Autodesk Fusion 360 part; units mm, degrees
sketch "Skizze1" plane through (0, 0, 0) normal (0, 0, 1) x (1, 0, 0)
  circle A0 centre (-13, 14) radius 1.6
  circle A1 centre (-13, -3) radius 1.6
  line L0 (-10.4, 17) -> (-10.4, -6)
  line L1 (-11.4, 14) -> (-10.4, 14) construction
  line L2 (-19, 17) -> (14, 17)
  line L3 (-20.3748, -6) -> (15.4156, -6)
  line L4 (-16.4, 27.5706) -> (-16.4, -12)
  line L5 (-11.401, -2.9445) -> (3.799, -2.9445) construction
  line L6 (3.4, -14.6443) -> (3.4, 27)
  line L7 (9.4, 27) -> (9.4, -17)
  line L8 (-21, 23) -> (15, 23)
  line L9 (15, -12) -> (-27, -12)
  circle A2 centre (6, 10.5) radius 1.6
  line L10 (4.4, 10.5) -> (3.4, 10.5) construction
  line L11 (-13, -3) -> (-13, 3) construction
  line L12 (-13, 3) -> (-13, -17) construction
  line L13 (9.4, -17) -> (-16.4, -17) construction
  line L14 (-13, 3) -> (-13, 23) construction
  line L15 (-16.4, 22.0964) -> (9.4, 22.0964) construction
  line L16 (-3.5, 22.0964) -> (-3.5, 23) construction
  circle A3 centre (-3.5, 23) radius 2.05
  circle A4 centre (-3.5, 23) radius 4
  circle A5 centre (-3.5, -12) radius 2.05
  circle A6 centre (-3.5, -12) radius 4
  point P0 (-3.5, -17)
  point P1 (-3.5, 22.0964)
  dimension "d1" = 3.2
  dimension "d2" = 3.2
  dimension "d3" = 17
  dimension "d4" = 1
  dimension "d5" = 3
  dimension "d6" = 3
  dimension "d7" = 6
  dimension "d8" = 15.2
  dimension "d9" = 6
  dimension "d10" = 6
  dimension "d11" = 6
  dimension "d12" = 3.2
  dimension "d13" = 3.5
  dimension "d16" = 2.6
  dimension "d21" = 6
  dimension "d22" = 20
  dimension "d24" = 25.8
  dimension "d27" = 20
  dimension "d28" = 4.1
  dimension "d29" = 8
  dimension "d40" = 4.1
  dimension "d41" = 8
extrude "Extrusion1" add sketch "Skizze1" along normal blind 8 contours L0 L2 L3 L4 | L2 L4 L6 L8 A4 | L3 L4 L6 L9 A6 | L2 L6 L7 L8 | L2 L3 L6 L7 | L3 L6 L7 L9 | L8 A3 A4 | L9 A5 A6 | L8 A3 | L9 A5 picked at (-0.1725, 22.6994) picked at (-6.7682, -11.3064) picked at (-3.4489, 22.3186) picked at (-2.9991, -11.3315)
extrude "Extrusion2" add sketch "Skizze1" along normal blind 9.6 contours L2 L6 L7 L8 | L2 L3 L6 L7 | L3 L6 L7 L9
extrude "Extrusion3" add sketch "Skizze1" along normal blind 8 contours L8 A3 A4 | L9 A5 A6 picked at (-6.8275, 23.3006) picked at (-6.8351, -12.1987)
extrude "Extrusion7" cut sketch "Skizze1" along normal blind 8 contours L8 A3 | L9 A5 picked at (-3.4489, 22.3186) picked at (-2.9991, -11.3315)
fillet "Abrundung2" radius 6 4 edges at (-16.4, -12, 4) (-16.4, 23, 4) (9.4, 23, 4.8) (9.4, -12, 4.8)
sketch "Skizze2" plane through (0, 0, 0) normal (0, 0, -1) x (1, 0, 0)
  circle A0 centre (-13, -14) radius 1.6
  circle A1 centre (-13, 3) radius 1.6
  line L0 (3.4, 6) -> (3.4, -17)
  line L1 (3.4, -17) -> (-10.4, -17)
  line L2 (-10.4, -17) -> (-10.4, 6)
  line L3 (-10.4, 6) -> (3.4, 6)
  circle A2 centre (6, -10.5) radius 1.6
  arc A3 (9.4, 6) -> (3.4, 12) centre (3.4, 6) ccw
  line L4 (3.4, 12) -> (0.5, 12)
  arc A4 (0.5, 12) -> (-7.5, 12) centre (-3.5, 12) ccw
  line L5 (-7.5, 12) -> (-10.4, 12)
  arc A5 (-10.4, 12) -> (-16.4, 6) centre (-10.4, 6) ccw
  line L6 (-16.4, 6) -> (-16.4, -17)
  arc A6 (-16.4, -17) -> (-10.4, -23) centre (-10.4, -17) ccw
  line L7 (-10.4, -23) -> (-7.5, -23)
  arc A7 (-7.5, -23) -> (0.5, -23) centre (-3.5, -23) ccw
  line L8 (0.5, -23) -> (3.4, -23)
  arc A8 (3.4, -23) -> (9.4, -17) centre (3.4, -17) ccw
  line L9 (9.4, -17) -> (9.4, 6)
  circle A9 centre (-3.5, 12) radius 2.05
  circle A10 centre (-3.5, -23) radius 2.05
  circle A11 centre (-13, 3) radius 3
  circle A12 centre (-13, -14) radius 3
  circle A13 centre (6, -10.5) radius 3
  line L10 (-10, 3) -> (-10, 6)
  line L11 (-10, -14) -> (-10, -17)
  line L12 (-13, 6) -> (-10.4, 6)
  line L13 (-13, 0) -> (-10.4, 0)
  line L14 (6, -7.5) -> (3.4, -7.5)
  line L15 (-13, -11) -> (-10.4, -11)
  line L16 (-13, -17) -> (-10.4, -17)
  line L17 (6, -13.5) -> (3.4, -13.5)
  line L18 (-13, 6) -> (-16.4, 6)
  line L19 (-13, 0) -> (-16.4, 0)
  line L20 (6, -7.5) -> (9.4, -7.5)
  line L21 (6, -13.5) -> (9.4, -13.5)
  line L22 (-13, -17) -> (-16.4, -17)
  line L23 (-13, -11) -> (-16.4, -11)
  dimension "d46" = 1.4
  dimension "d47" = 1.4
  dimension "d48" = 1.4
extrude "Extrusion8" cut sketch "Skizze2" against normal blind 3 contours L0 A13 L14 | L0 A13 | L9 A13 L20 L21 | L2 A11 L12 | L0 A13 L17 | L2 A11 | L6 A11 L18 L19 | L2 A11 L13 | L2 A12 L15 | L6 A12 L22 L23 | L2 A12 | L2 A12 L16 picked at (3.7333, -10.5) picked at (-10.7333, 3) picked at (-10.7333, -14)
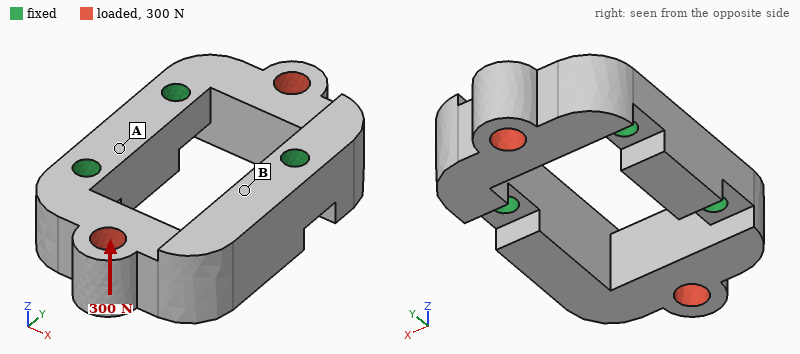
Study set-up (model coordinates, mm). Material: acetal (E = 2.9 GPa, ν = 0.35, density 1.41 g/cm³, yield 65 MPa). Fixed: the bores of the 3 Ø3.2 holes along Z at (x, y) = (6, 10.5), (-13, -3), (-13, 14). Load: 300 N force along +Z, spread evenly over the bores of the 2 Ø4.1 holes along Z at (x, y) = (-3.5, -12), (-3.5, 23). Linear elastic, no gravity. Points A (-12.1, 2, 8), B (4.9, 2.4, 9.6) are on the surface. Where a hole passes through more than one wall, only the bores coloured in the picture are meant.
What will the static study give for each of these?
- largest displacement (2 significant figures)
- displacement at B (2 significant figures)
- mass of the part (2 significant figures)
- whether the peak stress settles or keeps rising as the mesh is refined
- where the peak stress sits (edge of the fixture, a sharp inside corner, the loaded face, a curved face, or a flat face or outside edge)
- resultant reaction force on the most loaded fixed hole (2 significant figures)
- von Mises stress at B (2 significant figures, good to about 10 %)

0.33 mm
0.069 mm
6.3 g
keeps rising
edge of the fixture
120 N
9.2 MPa
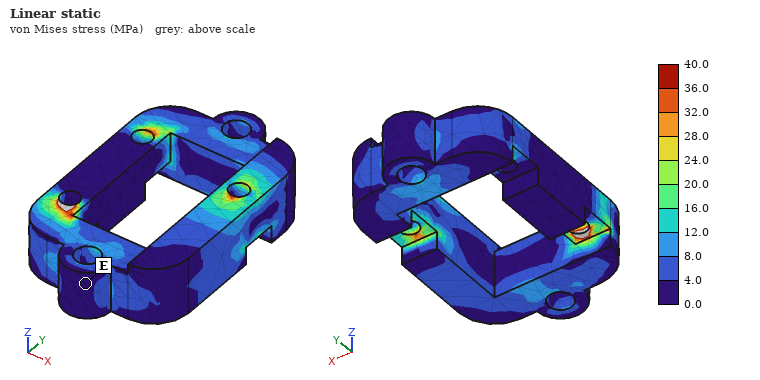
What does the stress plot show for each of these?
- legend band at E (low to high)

0.0 to 4.0 MPa
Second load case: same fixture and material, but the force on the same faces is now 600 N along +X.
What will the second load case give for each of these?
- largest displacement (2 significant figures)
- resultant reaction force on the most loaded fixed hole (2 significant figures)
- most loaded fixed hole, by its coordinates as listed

0.10 mm
280 N
(-13, -3)
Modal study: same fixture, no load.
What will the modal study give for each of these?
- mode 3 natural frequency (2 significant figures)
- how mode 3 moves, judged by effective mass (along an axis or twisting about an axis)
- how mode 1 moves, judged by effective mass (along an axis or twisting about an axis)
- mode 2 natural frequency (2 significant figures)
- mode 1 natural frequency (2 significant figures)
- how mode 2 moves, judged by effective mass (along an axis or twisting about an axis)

6700 Hz
along X
along Z
5500 Hz
3100 Hz
along Z
